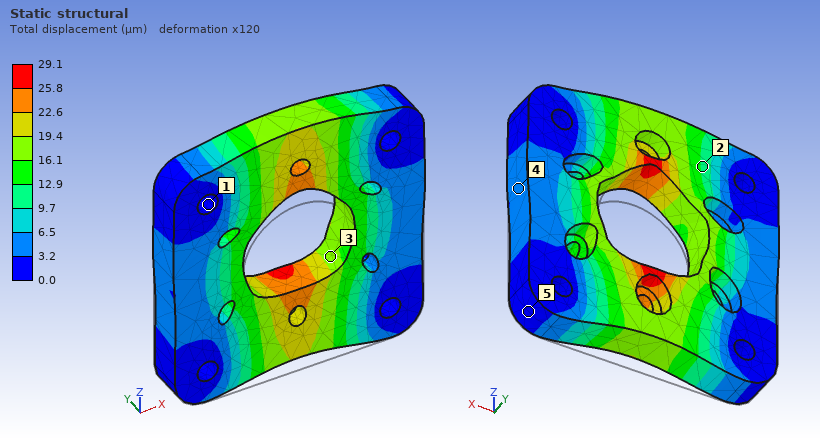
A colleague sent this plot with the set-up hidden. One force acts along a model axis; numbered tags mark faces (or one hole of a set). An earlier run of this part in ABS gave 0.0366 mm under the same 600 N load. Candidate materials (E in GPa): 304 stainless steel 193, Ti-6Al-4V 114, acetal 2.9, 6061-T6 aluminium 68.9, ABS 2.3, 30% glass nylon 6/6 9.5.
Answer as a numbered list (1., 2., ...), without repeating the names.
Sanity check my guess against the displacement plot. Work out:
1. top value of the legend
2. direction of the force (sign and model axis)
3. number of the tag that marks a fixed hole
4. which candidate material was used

1. 29.1 µm
2. +Z
3. 1
4. acetal
